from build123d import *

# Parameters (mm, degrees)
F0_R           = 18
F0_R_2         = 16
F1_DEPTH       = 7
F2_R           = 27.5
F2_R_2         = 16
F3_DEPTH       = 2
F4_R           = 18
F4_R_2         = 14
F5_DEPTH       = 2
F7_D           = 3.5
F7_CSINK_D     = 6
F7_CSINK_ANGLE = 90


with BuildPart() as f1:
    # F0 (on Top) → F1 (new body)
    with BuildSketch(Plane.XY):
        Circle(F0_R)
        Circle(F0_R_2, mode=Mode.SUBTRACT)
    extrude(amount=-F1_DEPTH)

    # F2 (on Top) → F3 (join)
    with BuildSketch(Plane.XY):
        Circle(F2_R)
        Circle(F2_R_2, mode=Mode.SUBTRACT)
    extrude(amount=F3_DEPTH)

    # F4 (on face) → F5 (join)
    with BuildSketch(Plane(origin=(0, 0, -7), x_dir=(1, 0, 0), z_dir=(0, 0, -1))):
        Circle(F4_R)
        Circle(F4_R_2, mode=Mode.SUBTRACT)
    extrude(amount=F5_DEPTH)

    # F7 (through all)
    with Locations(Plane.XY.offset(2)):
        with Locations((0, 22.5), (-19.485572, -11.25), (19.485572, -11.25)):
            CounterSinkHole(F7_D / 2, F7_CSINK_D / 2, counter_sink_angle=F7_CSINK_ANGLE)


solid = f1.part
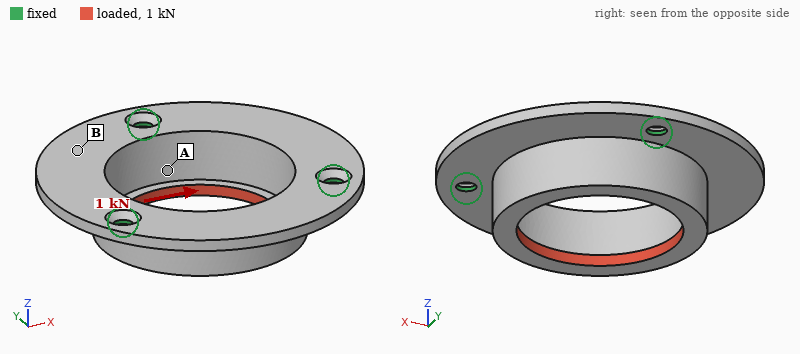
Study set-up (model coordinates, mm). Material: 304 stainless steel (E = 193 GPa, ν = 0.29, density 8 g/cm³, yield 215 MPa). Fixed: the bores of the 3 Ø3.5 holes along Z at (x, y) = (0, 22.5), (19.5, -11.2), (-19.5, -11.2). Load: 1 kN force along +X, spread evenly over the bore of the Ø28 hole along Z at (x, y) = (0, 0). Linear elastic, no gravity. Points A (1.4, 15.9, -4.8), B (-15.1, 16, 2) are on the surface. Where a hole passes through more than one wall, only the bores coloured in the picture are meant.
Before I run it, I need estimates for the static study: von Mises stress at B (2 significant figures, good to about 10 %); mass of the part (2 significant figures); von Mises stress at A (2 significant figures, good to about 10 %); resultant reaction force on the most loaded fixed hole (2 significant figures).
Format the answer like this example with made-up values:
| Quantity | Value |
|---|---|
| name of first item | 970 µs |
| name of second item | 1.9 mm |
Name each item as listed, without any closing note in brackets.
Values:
| Quantity | Value |
|---|---|
| von Mises stress at B | 14 MPa |
| mass of the part | 43 g |
| von Mises stress at A | 34 MPa |
| resultant reaction force on the most loaded fixed hole | 400 N |
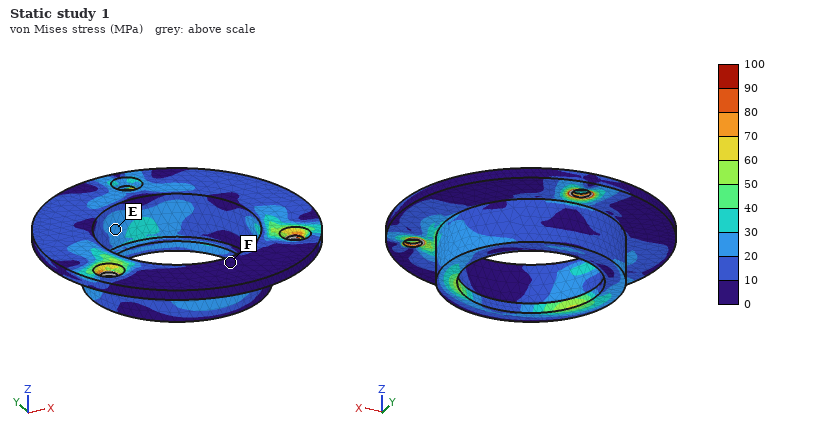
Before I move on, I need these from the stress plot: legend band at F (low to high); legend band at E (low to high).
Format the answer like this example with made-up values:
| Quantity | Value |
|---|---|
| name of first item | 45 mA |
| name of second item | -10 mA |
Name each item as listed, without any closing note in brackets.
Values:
| Quantity | Value |
|---|---|
| legend band at F | 0 to 10 MPa |
| legend band at E | 20 to 30 MPa |
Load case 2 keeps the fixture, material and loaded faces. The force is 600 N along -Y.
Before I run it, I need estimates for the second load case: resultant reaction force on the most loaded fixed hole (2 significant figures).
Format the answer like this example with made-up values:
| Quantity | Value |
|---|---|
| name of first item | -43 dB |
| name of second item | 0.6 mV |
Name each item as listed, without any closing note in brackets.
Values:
| Quantity | Value |
|---|---|
| resultant reaction force on the most loaded fixed hole | 240 N |
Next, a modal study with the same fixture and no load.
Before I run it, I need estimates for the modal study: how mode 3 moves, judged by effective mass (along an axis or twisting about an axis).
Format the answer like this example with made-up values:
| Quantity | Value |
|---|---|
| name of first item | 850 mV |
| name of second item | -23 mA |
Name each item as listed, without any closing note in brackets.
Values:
| Quantity | Value |
|---|---|
| how mode 3 moves, judged by effective mass | along Z |
